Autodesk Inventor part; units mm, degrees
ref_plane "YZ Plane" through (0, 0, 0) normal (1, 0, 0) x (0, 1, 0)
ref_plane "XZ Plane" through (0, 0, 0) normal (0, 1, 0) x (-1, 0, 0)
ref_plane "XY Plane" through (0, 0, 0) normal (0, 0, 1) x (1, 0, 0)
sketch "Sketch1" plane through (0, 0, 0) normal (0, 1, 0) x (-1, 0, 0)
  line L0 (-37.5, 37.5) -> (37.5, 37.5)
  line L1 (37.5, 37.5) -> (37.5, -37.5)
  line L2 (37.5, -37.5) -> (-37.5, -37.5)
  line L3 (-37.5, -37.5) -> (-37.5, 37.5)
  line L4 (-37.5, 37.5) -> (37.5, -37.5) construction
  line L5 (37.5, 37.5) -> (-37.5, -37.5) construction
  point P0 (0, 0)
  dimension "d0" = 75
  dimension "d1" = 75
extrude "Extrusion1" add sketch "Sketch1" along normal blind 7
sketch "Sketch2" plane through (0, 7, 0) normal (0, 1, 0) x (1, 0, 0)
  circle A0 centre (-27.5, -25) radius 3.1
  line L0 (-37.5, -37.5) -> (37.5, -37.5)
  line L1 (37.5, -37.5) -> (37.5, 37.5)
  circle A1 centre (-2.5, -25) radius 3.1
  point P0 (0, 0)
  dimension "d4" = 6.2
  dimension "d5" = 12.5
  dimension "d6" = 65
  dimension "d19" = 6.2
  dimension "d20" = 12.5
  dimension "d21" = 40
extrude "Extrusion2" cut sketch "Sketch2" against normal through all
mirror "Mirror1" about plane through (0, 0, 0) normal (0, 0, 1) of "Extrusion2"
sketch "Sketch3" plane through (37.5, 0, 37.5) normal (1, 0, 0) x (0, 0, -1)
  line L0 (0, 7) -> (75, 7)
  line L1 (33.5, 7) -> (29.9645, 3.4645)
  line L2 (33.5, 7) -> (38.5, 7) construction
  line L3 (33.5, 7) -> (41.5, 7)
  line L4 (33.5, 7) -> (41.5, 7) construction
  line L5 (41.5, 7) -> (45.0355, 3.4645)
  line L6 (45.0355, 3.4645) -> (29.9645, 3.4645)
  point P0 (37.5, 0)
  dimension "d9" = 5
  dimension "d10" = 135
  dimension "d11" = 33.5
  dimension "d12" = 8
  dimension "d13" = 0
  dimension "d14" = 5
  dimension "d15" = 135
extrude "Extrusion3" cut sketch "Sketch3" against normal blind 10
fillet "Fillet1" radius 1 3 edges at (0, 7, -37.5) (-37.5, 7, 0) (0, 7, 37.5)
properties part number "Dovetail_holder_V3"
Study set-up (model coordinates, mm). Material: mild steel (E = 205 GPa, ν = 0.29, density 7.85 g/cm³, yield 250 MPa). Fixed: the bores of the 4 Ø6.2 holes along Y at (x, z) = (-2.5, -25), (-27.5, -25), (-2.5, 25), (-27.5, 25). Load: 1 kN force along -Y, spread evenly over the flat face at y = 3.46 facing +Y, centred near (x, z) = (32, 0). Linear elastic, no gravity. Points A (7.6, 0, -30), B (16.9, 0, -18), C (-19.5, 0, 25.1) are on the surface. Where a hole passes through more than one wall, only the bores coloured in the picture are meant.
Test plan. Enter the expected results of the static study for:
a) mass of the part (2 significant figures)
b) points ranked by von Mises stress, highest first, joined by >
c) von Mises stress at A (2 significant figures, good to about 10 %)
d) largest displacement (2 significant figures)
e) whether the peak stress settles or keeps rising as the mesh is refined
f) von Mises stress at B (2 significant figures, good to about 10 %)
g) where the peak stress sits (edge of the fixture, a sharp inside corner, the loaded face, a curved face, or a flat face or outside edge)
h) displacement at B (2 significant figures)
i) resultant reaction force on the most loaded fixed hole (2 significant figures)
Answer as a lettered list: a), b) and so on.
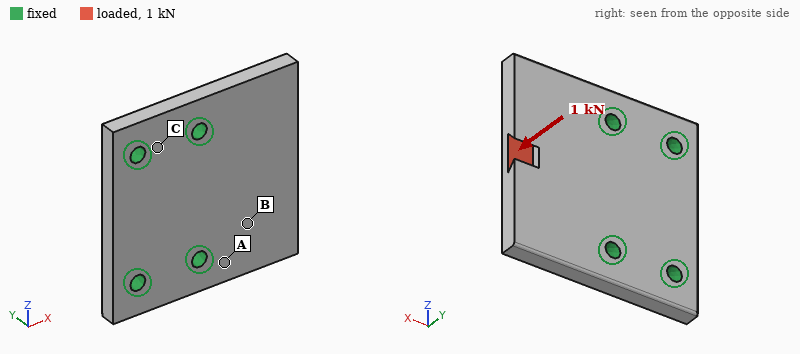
a) 300 g
b) A > B > C
c) 44 MPa
d) 59 µm
e) keeps rising
f) 26 MPa
g) edge of the fixture
h) 17 µm
i) 740 N
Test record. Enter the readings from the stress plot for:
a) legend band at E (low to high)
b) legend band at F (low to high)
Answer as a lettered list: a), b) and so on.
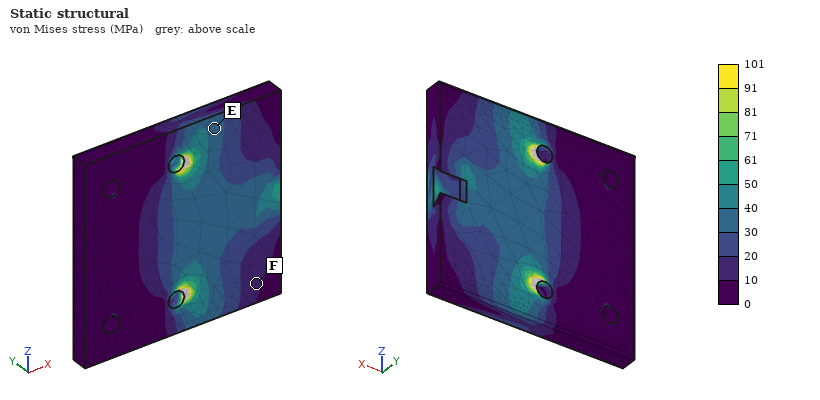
a) 30 to 40 MPa
b) 10 to 20 MPa
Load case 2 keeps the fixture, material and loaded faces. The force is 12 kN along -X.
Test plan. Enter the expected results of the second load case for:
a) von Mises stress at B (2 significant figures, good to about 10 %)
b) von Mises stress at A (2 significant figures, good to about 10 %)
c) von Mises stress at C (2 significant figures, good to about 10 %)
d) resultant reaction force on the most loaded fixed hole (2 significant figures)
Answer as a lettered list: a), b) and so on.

a) 37 MPa
b) 15 MPa
c) 9.3 MPa
d) 4.7 kN
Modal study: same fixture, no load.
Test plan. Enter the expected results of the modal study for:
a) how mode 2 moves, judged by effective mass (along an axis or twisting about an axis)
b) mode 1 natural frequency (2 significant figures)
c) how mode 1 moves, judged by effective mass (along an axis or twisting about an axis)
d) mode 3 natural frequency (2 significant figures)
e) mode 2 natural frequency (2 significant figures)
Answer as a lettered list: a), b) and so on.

a) twisting about X
b) 3400 Hz
c) along Y
d) 9400 Hz
e) 5400 Hz
